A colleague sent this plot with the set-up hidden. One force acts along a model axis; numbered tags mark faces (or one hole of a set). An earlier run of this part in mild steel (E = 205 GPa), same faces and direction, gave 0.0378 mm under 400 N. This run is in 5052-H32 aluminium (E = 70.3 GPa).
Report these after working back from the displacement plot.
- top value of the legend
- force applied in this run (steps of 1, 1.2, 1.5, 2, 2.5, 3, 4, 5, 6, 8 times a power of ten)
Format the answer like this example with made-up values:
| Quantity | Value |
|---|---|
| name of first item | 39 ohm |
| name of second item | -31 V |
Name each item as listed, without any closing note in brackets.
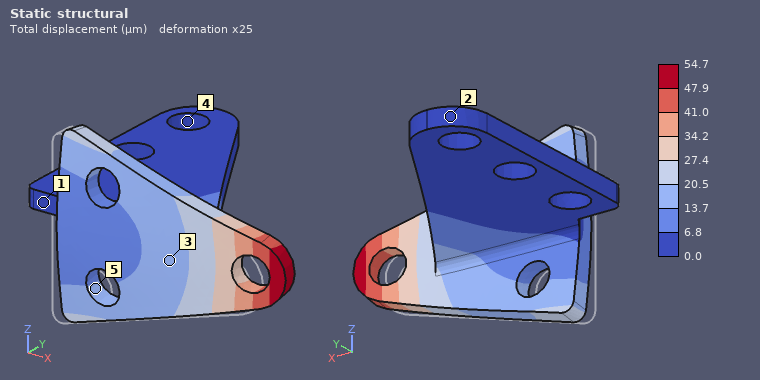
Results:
| Quantity | Value |
|---|---|
| top value of the legend | 54.7 µm |
| force applied in this run | 200 N |
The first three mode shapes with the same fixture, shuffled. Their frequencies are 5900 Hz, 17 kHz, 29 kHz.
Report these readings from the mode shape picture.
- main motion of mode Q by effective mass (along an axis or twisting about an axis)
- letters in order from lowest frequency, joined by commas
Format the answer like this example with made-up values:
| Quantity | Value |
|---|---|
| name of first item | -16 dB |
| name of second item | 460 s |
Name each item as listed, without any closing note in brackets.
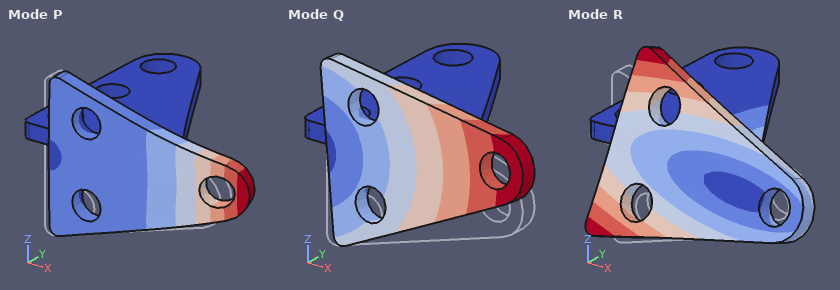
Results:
| Quantity | Value |
|---|---|
| main motion of mode Q by effective mass | along Z |
| letters in order from lowest frequency, joined by commas | Q, R, P |
